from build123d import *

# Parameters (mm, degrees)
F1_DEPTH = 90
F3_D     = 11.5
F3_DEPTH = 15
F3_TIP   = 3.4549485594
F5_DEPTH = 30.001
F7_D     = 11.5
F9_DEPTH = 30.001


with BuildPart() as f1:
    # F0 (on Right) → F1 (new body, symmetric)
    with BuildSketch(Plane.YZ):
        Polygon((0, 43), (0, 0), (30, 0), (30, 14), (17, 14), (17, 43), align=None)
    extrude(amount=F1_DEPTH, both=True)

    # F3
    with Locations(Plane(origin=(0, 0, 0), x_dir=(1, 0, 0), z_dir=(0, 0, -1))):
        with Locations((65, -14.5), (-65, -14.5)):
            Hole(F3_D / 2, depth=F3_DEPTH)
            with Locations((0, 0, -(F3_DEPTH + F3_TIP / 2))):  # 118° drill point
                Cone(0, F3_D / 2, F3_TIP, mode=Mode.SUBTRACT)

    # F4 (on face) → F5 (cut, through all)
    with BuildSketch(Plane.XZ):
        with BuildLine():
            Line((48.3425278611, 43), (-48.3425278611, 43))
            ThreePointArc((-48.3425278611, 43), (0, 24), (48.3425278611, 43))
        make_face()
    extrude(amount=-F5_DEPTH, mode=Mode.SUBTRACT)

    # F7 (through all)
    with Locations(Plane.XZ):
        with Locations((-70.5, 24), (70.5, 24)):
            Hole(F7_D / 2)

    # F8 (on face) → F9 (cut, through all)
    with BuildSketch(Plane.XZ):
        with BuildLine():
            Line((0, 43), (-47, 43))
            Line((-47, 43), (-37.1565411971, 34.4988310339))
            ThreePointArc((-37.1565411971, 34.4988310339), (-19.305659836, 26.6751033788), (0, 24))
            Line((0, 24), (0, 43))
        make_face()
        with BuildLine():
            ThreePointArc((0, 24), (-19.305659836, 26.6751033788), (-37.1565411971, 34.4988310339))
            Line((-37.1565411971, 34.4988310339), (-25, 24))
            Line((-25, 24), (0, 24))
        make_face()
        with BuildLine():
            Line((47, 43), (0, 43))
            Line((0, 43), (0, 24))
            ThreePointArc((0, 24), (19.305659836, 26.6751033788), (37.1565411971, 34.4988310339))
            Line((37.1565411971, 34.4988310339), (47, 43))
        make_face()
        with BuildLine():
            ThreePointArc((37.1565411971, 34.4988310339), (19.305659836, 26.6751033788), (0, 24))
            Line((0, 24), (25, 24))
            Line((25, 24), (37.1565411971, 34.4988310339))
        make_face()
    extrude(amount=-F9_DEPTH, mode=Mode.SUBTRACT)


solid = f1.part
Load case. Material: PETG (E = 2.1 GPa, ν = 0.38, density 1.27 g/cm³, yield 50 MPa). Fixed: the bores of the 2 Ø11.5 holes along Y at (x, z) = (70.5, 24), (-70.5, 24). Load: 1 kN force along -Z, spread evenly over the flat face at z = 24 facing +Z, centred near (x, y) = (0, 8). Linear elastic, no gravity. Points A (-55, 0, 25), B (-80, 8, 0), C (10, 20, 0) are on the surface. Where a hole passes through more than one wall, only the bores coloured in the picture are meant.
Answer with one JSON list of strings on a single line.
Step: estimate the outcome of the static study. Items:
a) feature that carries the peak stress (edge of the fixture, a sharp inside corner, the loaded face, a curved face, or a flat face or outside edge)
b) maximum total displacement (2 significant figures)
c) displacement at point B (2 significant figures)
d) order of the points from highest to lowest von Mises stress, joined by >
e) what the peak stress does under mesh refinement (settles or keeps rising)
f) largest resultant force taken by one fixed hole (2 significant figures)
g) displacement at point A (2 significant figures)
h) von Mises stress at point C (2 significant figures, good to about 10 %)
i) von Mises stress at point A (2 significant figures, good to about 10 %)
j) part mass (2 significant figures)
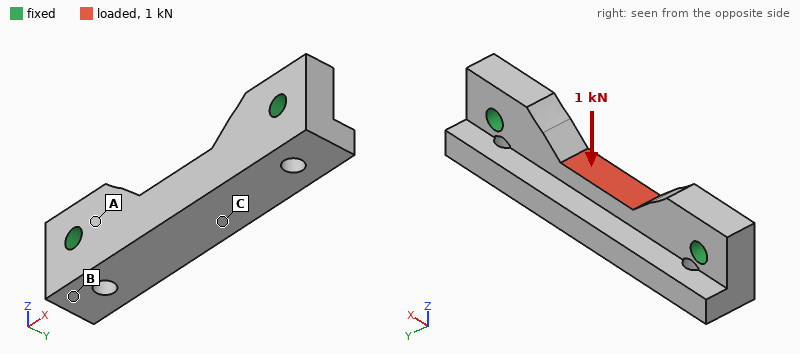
["edge of the fixture", "0.25 mm", "0.045 mm", "C > A > B", "keeps rising", "790 N", "0.042 mm", "3.7 MPa", "1.9 MPa", "170 g"]
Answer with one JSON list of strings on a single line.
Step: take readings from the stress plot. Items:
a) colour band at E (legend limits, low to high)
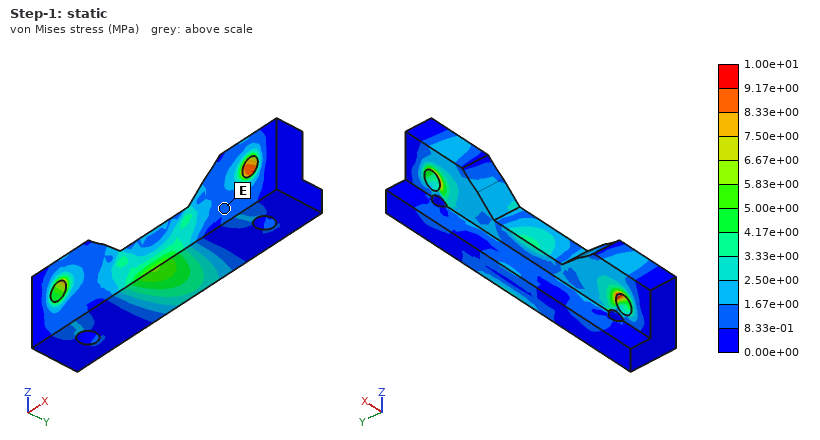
["8.33e-01 to 1.67e+00 MPa"]
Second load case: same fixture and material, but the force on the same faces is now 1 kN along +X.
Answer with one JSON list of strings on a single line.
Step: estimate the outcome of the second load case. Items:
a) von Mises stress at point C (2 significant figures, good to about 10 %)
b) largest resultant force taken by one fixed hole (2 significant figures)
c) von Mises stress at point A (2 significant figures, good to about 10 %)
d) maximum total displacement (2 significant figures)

["0.55 MPa", "500 N", "1.3 MPa", "59 µm"]
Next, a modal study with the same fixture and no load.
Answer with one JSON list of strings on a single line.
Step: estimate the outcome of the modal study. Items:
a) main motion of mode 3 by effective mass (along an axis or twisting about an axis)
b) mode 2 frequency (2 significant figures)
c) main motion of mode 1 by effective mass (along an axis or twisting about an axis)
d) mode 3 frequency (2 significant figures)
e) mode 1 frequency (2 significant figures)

["twisting about X", "1500 Hz", "along Y", "2200 Hz", "1100 Hz"]
